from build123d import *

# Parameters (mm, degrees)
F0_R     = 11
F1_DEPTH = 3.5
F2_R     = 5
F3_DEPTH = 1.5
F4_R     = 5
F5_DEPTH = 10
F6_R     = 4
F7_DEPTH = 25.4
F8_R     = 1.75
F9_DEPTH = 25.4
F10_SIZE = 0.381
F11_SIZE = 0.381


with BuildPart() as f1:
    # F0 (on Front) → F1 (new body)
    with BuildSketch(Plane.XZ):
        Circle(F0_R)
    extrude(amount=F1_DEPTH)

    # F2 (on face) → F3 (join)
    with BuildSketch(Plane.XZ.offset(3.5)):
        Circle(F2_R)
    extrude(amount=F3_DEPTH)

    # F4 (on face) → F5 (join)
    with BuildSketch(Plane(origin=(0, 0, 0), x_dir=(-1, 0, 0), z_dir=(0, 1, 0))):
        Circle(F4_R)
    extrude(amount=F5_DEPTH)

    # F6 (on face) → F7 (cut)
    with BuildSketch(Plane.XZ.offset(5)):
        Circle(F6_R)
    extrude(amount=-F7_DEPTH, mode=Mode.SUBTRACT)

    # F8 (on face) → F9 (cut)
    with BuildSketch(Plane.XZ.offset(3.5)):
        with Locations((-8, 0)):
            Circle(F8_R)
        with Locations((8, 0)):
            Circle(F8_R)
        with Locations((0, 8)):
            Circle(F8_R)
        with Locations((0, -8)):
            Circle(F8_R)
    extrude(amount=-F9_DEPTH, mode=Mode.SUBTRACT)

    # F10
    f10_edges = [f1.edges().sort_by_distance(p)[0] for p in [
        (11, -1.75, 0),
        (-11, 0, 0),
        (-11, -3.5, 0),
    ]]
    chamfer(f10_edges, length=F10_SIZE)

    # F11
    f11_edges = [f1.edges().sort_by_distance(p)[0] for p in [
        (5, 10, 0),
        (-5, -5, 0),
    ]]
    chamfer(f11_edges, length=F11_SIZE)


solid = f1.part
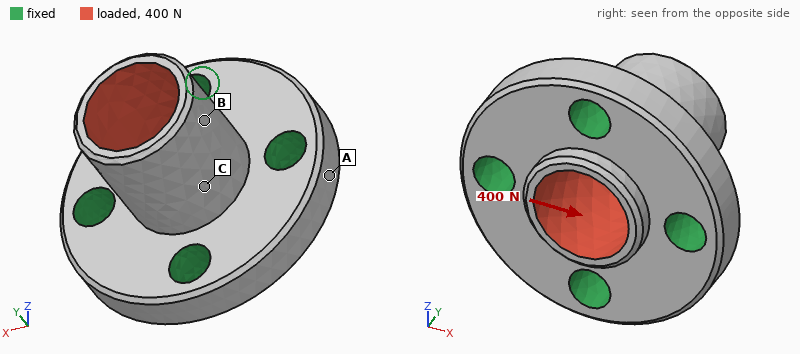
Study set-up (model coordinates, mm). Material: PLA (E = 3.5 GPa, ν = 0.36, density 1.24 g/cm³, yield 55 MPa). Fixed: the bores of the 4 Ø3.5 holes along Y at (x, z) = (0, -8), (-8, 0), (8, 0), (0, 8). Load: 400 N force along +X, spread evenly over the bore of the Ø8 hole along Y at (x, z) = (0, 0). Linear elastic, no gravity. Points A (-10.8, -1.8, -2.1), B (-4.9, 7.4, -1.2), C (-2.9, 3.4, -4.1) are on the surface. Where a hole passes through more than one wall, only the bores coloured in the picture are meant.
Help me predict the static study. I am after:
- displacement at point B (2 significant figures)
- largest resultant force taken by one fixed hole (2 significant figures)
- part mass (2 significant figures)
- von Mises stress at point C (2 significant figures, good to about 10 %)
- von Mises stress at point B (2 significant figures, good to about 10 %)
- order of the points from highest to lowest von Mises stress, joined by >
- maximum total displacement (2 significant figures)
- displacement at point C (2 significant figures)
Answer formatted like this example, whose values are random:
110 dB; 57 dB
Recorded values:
0.13 mm; 170 N; 1.6 g; 16 MPa; 5.3 MPa; C > B > A; 0.15 mm; 0.067 mm
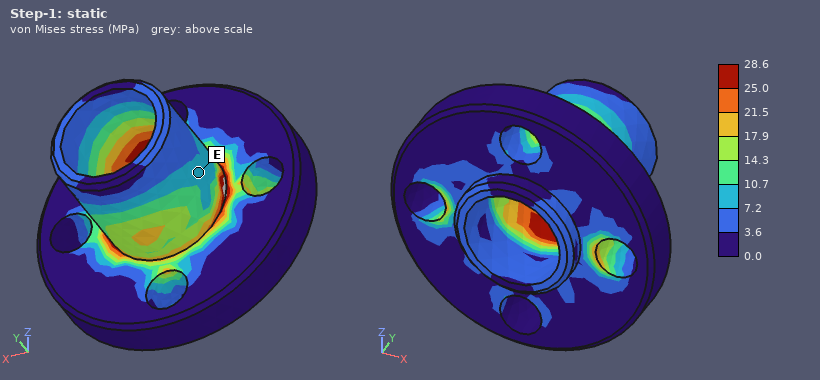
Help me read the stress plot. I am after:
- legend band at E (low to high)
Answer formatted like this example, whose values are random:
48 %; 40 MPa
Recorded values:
7.2 to 10.7 MPa
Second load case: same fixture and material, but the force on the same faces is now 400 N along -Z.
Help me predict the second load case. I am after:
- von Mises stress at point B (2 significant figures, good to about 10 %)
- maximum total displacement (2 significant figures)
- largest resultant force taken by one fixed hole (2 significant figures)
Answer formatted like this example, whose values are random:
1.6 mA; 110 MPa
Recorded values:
8.0 MPa; 0.15 mm; 170 N
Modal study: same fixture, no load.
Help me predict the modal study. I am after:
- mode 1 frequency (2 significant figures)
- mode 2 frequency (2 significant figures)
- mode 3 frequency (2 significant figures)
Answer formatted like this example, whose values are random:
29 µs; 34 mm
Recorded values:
13 kHz; 13 kHz; 13 kHz
